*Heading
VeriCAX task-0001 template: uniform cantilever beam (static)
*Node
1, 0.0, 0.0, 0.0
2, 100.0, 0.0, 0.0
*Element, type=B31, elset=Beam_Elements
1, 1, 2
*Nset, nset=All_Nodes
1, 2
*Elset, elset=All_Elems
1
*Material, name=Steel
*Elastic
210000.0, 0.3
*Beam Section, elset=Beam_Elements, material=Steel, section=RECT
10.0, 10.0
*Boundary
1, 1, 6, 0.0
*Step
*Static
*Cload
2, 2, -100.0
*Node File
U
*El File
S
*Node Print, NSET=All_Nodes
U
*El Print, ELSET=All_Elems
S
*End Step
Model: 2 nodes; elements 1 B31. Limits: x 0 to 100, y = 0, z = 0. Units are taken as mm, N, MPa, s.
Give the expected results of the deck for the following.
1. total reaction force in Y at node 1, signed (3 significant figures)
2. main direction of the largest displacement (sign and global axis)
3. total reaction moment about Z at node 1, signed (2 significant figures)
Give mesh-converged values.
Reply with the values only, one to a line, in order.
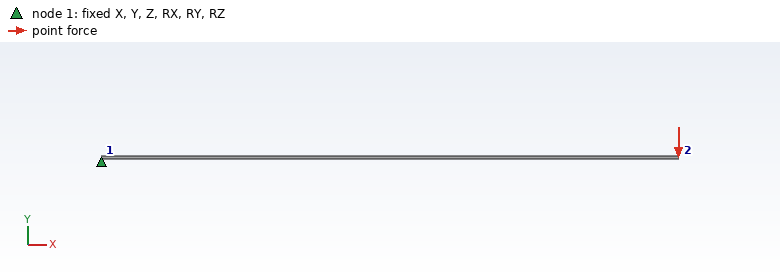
100 N
-Y
10000 N·mm
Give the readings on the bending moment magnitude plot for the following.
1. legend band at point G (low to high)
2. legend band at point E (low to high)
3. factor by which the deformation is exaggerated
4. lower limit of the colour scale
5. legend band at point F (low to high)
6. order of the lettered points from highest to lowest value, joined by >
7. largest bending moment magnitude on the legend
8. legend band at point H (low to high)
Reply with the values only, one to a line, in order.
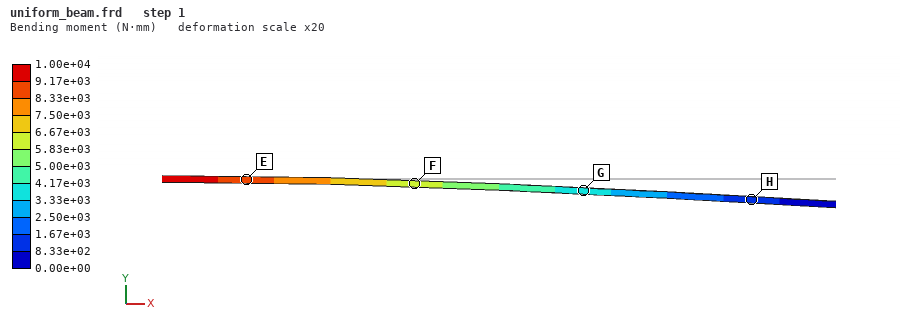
3.33e+03 to 4.17e+03 N·mm
8.33e+03 to 9.17e+03 N·mm
20
0.00e+00 N·mm
5.83e+03 to 6.67e+03 N·mm
E > F > G > H
1.00e+04 N·mm
8.33e+02 to 1.67e+03 N·mm
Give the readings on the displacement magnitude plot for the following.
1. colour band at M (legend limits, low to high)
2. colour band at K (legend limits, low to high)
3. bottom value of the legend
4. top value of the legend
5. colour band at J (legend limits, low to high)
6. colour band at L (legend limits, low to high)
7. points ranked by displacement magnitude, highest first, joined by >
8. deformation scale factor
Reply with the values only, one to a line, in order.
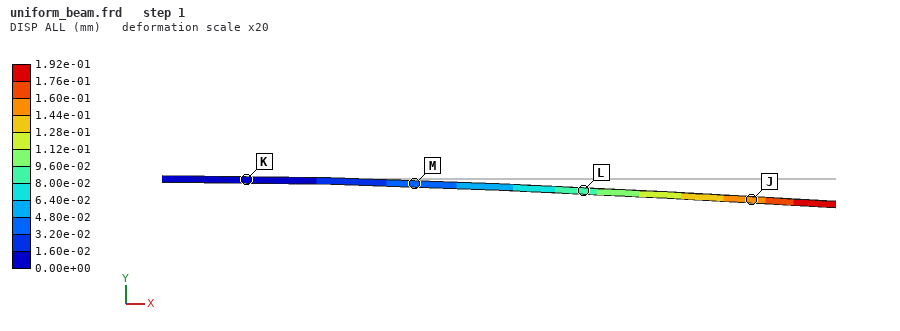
3.20e-02 to 4.80e-02 mm
0.00e+00 to 1.60e-02 mm
0.00e+00 mm
1.92e-01 mm
1.44e-01 to 1.60e-01 mm
8.00e-02 to 9.60e-02 mm
J > L > M > K
20
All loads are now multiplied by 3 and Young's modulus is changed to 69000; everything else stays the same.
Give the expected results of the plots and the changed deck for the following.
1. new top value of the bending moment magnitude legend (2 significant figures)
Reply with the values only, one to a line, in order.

30000 N·mm
